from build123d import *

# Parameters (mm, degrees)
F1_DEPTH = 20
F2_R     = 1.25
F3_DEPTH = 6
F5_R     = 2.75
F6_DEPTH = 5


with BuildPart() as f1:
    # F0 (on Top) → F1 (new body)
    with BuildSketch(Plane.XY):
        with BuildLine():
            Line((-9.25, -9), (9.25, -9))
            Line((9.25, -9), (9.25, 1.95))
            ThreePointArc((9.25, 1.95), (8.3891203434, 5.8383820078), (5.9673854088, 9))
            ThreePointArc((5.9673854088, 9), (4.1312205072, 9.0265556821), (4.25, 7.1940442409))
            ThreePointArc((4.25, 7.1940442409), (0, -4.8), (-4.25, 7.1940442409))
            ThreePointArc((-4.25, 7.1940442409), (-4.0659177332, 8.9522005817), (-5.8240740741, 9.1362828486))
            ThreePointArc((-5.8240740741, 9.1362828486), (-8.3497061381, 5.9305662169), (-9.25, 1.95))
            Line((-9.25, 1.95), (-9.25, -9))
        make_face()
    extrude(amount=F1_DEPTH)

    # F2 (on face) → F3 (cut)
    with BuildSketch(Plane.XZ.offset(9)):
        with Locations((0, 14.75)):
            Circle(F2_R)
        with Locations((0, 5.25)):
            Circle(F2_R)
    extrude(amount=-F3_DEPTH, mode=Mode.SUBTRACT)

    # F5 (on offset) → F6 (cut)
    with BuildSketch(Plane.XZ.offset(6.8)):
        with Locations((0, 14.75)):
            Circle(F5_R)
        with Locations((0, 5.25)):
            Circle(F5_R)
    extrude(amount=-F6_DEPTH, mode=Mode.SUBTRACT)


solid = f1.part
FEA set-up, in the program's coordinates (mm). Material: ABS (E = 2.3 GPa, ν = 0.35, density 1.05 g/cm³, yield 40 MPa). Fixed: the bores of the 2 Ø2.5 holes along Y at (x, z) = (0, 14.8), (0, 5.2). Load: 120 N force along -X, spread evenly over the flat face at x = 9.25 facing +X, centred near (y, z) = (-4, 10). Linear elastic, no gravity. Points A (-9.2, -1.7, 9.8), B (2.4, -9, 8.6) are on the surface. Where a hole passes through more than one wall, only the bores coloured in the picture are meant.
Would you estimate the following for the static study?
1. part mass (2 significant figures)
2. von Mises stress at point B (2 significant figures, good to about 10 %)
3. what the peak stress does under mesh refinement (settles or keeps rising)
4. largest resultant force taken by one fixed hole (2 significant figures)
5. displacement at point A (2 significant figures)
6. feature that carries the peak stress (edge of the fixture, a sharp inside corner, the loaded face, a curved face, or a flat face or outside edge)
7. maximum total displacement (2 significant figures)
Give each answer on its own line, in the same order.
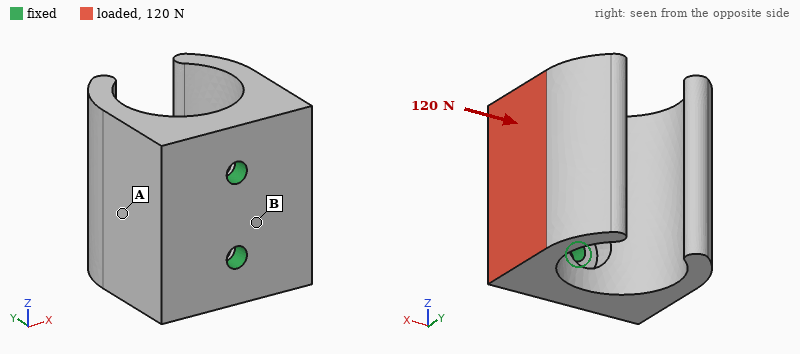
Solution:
3.5 g
6.4 MPa
keeps rising
60 N
0.11 mm
edge of the fixture
0.34 mm
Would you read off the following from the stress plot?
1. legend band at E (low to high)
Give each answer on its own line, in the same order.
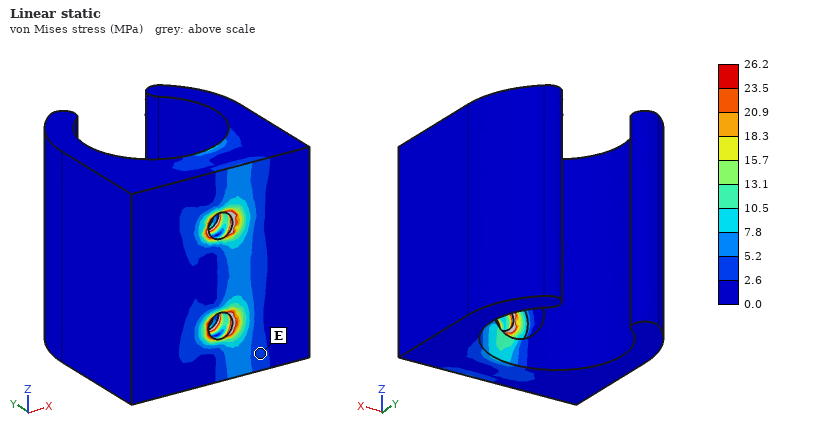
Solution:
2.6 to 5.2 MPa
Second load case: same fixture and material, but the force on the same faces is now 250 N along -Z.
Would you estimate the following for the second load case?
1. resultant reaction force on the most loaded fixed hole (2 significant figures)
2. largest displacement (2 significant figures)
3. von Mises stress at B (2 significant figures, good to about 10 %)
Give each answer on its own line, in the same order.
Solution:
260 N
0.16 mm
7.5 MPa
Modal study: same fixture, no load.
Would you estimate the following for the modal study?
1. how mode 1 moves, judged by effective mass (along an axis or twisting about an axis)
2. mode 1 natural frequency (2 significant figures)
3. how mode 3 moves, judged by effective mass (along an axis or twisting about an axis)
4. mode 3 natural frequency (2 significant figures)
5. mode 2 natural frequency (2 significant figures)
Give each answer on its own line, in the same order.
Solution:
along X
1700 Hz
along Z
3800 Hz
2800 Hz
